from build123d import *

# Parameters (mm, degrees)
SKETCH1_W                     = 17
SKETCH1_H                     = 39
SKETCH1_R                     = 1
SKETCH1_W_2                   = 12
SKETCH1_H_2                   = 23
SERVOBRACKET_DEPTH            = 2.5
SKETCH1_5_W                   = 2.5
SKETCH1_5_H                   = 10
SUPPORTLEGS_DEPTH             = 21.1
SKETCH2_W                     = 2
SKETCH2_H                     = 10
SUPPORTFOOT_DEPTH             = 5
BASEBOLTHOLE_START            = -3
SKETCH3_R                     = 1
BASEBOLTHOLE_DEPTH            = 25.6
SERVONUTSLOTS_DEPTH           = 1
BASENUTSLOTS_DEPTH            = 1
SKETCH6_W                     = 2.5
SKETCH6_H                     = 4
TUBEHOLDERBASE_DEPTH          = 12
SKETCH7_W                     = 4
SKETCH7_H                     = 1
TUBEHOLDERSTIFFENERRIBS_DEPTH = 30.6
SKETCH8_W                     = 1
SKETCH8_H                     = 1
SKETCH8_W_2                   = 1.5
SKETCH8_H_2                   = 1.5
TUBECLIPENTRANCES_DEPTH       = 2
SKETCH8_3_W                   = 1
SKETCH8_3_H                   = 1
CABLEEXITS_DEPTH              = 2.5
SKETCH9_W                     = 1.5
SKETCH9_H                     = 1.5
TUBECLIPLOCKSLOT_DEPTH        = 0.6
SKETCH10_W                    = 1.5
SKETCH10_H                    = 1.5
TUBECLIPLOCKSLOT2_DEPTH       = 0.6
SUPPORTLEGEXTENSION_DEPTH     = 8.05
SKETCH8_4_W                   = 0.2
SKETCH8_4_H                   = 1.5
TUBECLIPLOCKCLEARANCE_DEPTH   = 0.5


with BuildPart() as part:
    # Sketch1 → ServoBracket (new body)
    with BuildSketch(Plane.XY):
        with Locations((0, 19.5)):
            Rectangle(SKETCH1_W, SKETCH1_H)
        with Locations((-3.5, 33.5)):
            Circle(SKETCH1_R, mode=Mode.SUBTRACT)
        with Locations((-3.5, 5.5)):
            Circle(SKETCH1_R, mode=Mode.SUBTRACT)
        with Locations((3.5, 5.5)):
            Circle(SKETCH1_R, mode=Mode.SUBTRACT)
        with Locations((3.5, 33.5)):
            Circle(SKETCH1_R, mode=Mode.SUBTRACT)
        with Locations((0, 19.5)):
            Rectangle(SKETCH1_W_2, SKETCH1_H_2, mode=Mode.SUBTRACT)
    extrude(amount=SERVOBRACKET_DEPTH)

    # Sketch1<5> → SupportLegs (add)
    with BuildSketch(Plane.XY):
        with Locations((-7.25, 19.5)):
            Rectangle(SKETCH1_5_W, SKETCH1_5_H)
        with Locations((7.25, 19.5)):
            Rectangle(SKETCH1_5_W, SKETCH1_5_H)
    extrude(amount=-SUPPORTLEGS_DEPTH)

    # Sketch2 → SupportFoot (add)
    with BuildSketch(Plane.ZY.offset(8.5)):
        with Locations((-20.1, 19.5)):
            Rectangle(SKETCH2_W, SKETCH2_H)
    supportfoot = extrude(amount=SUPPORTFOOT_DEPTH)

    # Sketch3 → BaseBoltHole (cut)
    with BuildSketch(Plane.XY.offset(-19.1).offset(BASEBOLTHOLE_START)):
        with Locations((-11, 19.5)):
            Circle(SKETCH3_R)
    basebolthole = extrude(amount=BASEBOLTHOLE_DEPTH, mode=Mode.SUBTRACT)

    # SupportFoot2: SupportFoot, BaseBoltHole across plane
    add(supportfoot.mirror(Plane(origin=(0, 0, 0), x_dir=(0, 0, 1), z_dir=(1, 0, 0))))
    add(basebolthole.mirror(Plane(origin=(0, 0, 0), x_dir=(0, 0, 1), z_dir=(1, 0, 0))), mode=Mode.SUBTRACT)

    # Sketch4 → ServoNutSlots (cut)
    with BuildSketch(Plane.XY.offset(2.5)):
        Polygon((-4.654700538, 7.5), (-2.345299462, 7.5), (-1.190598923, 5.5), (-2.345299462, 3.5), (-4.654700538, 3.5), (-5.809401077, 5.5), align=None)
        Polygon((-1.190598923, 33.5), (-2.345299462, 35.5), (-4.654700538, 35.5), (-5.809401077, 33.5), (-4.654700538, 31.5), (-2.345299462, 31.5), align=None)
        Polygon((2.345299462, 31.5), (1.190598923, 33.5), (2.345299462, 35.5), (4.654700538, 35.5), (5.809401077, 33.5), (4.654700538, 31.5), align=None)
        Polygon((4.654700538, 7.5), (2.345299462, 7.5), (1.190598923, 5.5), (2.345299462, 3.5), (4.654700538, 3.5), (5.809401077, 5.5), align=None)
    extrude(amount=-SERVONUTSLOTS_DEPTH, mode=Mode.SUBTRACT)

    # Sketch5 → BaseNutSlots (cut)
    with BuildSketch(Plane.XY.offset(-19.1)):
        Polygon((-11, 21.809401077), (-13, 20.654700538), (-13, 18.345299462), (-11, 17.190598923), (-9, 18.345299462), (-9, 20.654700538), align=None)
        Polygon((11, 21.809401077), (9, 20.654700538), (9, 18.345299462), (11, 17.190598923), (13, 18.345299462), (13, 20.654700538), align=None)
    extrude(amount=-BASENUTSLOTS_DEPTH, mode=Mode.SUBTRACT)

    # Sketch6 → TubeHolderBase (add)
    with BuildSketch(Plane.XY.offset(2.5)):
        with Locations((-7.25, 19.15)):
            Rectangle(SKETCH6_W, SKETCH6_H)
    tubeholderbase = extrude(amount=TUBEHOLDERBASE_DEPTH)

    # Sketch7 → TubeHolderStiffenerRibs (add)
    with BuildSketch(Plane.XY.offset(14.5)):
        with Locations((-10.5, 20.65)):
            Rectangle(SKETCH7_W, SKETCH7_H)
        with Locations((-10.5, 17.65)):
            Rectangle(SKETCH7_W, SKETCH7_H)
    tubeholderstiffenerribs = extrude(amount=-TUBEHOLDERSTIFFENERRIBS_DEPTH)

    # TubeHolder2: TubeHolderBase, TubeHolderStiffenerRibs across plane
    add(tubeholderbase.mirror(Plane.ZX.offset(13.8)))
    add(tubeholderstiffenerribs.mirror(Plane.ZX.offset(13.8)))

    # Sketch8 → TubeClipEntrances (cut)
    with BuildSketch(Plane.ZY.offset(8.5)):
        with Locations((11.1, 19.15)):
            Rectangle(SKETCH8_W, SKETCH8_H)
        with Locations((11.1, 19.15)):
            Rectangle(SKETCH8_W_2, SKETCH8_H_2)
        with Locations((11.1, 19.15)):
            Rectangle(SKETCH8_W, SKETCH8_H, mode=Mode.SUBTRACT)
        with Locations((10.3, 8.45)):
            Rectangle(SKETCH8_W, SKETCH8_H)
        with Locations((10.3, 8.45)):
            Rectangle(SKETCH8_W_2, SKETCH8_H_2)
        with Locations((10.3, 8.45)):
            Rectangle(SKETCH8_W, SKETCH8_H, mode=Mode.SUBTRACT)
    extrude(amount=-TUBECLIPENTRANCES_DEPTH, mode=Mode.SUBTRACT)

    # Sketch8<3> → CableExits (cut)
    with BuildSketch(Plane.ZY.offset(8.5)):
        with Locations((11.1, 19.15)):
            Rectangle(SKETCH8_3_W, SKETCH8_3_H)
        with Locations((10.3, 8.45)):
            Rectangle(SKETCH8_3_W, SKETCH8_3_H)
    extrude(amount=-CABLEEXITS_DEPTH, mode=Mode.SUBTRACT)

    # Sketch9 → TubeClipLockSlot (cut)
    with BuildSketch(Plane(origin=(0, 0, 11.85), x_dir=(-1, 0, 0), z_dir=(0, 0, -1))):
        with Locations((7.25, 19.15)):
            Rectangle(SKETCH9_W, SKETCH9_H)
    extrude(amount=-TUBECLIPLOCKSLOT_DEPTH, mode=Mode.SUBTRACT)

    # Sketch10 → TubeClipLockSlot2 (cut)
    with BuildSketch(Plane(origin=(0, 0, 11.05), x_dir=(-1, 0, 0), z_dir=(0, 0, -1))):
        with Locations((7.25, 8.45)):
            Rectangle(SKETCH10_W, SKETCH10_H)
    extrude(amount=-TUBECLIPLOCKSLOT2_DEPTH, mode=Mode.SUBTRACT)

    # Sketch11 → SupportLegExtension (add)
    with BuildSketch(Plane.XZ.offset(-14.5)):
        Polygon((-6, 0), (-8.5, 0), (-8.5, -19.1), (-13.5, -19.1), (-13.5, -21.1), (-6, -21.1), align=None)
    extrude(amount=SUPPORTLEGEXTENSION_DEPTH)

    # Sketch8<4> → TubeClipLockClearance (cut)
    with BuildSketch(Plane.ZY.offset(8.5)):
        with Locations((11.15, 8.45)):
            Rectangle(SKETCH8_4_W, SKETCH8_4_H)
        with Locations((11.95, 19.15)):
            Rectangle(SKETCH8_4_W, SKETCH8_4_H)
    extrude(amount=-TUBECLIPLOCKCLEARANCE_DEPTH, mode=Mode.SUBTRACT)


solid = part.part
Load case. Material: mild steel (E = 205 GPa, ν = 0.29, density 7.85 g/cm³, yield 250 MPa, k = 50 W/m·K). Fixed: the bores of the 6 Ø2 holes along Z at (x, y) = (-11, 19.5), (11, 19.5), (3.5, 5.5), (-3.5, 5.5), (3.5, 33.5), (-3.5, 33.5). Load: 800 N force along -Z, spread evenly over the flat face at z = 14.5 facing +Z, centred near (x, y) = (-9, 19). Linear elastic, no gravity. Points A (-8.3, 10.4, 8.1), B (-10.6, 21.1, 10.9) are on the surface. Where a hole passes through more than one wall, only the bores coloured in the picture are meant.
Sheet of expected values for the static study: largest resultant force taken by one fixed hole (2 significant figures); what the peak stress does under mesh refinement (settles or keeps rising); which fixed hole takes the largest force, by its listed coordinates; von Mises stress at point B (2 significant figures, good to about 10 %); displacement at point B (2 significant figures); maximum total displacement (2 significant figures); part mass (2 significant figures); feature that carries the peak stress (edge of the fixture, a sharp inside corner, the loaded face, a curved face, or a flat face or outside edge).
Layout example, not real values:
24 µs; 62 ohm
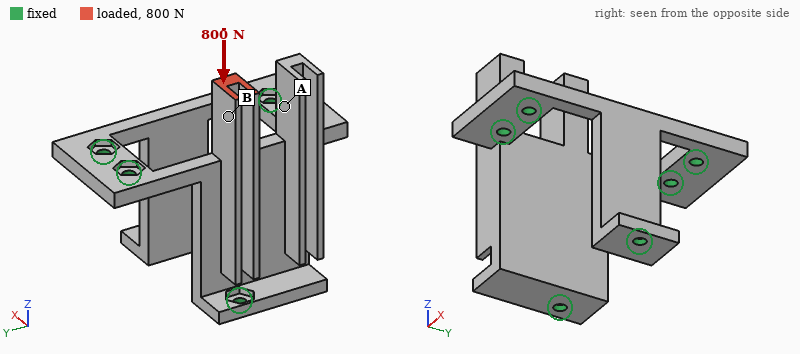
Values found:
470 N; keeps rising; (-11, 19.5); 43 MPa; 16 µm; 19 µm; 26 g; edge of the fixture
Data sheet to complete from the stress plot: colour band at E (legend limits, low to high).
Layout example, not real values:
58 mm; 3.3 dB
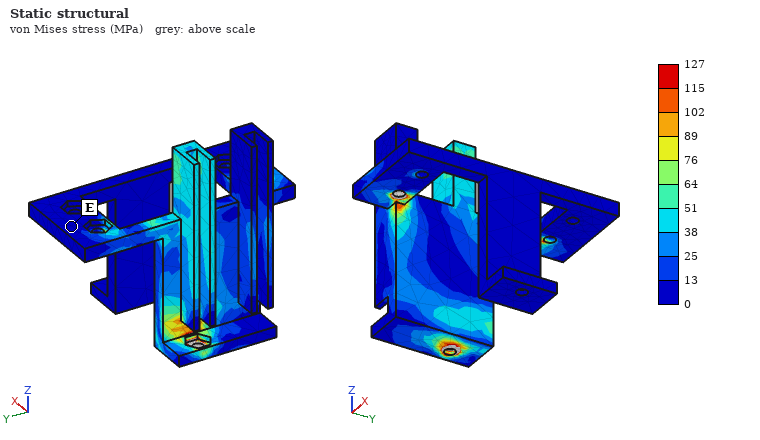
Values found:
0 to 13 MPa
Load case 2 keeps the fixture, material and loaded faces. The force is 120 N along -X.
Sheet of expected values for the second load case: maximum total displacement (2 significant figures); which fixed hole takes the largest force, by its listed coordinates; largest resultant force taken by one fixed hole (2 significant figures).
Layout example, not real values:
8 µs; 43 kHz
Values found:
44 µm; (-3.5, 5.5); 120 N
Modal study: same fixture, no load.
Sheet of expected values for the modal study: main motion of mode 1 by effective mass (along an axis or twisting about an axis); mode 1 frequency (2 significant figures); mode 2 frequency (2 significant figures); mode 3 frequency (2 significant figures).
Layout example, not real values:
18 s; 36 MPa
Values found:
along X; 7600 Hz; 9500 Hz; 10 kHz
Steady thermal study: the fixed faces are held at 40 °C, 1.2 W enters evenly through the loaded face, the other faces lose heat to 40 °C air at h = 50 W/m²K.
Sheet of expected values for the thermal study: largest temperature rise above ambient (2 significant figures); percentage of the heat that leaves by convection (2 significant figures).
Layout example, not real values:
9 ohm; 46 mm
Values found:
23 K; 47 %
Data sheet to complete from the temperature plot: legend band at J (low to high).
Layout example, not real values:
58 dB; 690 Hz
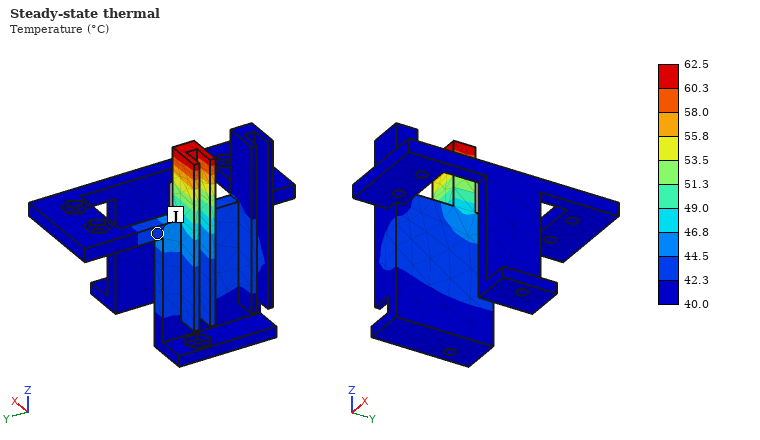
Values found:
42.3 to 44.5 °C
